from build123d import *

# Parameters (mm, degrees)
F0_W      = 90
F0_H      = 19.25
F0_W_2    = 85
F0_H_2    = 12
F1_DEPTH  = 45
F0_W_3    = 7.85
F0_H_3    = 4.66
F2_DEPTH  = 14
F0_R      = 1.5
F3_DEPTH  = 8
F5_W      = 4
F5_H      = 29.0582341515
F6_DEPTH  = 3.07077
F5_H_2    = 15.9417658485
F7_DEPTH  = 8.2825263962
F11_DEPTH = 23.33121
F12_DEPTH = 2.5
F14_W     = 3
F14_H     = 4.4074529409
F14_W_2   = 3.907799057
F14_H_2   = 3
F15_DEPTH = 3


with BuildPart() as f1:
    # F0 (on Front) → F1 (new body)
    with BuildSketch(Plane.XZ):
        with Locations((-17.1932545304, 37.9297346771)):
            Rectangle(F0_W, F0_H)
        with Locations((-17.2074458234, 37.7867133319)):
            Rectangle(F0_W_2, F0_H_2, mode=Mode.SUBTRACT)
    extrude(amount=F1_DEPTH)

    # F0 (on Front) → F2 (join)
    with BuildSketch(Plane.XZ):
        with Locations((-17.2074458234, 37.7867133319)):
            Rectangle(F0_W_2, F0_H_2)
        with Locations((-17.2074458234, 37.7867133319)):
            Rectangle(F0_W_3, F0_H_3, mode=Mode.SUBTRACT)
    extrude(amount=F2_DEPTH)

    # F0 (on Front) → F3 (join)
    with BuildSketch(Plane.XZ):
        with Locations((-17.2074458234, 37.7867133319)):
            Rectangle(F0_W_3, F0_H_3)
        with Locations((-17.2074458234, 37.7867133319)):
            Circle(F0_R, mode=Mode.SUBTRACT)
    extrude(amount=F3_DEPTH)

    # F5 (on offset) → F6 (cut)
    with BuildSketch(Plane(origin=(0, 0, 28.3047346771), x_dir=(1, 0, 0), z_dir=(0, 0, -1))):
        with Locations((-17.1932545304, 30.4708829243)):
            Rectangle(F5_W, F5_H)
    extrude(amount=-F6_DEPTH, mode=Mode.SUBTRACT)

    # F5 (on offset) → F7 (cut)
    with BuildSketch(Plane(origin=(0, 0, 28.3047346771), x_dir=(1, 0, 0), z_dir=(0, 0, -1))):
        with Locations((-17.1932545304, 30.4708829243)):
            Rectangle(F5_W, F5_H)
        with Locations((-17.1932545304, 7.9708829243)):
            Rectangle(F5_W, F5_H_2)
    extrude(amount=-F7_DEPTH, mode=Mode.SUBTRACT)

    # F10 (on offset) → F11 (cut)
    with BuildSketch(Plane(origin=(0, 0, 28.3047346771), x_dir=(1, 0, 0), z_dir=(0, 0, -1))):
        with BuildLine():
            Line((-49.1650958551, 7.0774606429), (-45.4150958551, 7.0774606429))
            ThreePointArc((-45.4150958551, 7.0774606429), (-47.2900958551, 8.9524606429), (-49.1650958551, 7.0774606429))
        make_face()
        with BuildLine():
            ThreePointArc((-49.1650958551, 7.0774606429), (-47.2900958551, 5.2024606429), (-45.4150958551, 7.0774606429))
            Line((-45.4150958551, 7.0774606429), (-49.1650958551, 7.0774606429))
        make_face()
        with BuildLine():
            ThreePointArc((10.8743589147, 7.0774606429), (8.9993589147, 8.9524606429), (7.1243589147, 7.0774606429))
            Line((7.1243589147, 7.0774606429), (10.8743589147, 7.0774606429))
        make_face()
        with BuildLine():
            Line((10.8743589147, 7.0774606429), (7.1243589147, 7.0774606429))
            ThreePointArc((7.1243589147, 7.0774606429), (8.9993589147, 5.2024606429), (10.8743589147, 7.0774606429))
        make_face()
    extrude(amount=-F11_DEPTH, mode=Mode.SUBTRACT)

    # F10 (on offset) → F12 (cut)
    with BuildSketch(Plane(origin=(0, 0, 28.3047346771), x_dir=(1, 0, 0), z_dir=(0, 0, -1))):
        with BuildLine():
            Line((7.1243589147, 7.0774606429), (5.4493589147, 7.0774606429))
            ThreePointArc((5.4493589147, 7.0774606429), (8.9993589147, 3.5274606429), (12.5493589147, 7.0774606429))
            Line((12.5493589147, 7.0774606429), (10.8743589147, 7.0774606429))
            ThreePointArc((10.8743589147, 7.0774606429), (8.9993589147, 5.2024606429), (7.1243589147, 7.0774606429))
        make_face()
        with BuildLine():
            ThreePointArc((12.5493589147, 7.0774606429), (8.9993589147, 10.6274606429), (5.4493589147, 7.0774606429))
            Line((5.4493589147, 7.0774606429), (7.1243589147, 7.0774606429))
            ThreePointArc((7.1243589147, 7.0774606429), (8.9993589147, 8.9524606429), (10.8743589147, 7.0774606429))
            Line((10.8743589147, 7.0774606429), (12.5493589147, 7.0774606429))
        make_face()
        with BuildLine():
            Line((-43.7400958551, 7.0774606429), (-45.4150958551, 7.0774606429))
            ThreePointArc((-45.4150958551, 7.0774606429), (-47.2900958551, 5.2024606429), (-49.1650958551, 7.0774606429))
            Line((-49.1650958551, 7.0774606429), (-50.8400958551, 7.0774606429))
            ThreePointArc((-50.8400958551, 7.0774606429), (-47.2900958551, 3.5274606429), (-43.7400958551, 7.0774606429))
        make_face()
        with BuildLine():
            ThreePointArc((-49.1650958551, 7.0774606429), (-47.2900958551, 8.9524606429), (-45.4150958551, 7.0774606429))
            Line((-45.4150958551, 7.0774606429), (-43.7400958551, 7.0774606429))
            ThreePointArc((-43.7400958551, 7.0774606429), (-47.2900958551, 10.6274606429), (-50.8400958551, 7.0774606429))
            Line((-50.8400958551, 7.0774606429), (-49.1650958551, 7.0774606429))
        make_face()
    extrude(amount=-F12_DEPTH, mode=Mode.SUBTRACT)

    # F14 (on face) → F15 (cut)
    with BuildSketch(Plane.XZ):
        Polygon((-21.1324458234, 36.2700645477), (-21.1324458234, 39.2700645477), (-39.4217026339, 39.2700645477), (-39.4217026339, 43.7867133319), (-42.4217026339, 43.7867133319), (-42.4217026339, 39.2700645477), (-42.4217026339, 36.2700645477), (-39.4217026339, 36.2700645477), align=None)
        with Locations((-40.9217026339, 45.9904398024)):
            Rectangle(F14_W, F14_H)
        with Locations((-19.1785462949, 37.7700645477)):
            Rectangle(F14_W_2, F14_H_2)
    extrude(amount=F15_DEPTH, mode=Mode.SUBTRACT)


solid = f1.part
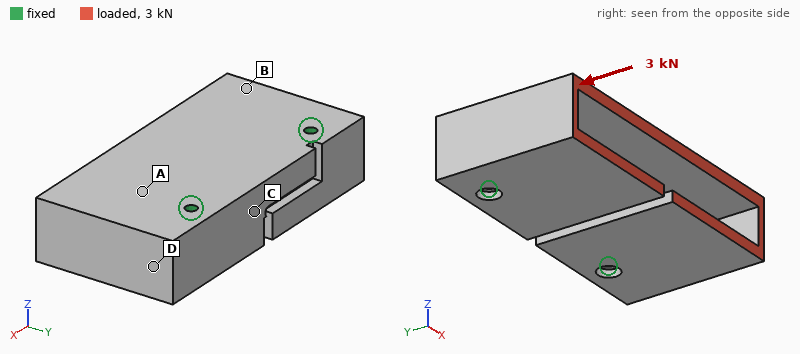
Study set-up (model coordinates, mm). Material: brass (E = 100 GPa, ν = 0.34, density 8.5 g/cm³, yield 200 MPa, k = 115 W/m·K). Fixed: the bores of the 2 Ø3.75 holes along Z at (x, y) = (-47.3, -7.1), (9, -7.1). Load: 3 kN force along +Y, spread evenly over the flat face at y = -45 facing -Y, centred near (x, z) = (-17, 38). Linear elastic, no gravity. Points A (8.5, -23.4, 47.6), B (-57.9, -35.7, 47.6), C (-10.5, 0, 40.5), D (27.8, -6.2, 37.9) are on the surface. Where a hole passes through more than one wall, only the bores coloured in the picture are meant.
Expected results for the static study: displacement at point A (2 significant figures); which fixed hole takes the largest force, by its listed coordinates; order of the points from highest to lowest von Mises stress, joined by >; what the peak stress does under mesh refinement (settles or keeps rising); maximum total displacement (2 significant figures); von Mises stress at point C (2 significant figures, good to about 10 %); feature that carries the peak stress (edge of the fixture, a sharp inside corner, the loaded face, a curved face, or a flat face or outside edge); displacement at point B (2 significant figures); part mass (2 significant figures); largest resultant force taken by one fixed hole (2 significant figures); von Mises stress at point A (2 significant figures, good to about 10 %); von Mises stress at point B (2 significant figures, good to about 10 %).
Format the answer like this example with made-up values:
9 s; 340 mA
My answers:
1.5 µm; (9, -7.1); A > B > C > D; keeps rising; 5.3 µm; 2.5 MPa; edge of the fixture; 1.7 µm; 380 g; 1.6 kN; 6.6 MPa; 4.7 MPa
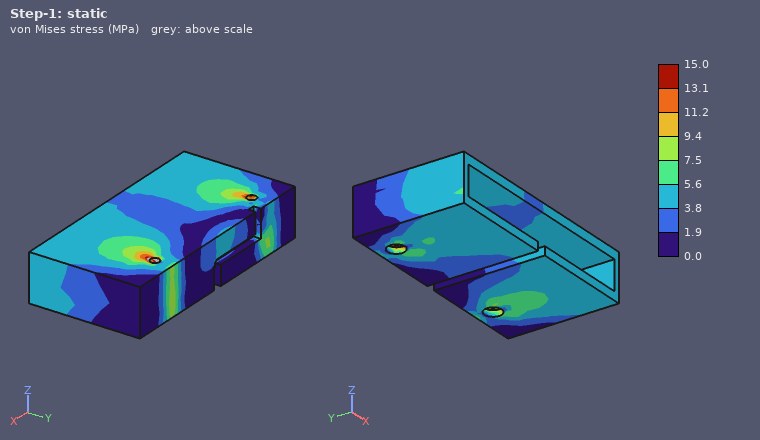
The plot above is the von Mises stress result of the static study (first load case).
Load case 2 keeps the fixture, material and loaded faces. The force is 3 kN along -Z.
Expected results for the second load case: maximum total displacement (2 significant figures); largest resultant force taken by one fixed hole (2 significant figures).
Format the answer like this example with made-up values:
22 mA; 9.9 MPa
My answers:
0.33 mm; 1.7 kN
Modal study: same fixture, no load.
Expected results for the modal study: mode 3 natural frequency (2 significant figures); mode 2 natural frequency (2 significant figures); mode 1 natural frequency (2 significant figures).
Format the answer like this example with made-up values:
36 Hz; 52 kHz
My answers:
2700 Hz; 2500 Hz; 2500 Hz
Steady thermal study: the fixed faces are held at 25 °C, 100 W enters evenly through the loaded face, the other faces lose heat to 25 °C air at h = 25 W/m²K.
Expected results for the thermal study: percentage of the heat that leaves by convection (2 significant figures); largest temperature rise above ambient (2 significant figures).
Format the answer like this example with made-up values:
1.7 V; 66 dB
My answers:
10 %; 48 K
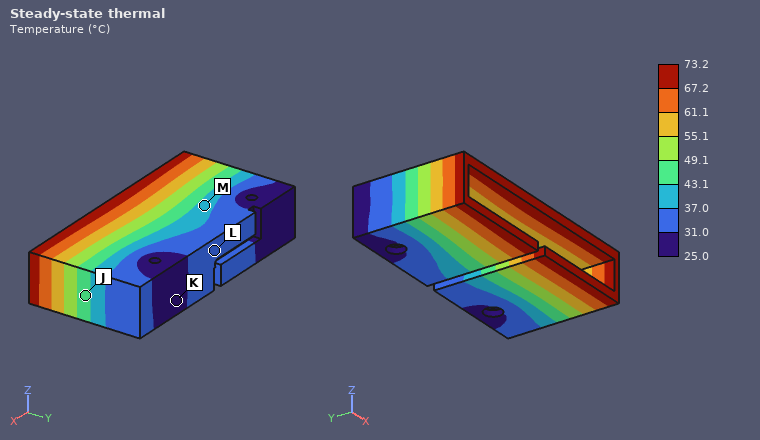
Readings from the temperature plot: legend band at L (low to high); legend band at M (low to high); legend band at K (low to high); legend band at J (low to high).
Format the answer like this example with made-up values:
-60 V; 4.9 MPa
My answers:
31.0 to 37.0 °C; 37.0 to 43.1 °C; 25.0 to 31.0 °C; 43.1 to 49.1 °C
